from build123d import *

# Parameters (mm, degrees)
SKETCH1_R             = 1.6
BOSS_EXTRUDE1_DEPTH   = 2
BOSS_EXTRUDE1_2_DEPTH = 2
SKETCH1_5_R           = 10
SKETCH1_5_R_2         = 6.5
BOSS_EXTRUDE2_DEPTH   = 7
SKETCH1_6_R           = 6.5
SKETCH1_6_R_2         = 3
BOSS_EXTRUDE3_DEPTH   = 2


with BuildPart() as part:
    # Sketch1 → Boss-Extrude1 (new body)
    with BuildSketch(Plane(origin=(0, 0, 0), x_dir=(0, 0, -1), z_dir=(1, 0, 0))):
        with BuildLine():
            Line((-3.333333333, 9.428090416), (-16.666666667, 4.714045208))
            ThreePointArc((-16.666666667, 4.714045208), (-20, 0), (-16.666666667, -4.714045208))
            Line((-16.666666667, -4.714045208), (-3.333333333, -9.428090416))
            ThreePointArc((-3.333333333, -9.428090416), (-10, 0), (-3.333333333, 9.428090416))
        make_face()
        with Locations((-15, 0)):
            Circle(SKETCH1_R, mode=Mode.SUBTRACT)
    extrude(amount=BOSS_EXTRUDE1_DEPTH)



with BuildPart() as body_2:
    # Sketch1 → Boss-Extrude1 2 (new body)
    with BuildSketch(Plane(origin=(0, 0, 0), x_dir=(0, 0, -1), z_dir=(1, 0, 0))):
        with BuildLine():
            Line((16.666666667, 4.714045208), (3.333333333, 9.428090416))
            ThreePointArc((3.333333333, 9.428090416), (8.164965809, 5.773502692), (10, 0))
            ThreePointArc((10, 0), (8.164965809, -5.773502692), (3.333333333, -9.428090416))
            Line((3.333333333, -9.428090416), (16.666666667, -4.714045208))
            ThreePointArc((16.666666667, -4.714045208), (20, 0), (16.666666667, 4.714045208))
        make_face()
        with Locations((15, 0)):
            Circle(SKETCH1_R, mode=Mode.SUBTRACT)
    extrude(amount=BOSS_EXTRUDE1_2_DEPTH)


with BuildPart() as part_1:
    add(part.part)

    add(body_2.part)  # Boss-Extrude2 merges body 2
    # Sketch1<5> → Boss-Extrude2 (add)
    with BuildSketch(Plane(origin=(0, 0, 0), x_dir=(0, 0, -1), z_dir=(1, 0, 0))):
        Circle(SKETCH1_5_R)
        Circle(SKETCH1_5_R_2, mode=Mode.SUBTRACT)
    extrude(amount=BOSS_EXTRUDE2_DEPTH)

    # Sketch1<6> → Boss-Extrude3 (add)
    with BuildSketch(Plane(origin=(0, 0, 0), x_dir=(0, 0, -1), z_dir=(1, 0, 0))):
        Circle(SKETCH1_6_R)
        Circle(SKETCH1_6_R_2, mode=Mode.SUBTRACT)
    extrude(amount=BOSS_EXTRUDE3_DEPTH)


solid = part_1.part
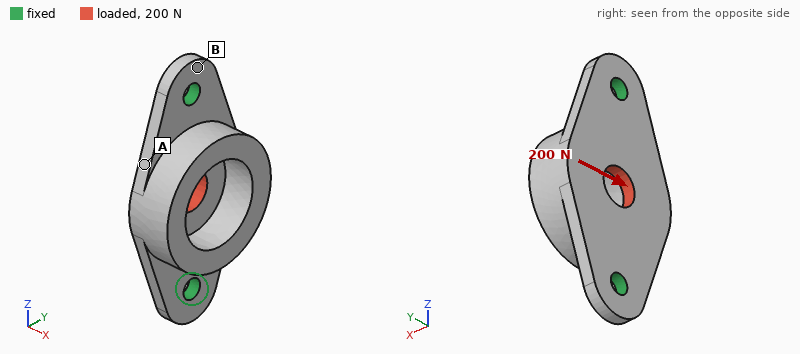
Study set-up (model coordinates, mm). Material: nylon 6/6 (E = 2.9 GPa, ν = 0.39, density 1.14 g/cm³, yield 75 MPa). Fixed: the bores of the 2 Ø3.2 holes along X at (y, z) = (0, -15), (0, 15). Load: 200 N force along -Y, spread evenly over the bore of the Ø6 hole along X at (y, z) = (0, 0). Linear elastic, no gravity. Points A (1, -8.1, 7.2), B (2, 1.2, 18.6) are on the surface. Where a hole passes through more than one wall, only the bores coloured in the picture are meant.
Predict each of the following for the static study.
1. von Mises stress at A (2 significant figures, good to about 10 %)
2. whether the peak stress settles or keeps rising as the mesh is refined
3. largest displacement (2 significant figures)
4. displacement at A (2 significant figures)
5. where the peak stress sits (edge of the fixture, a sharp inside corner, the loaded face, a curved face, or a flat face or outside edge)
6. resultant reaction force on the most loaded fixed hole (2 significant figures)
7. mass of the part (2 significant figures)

7.6 MPa
keeps rising
60 µm
40 µm
edge of the fixture
100 N
2.2 g
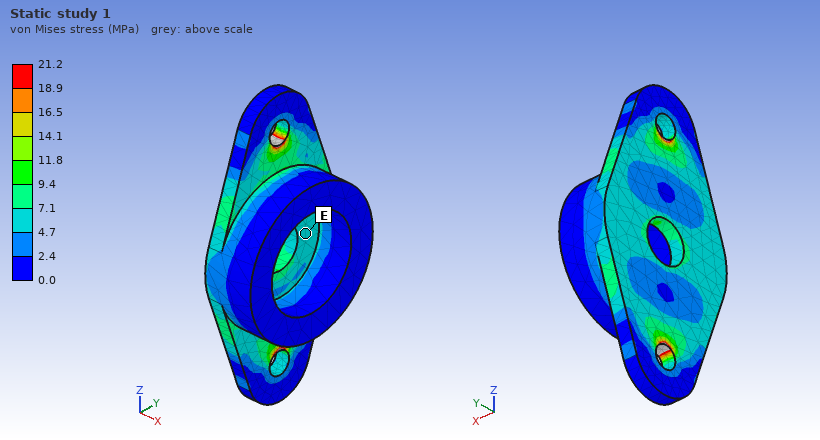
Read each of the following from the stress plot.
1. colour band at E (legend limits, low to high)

4.7 to 7.1 MPa
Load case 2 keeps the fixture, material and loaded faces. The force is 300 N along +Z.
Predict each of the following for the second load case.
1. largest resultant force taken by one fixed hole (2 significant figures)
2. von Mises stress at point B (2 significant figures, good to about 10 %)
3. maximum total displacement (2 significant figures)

150 N
2.9 MPa
35 µm
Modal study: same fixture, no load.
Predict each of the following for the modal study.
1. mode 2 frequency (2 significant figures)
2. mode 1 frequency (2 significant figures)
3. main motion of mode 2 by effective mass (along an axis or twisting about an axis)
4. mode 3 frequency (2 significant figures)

4100 Hz
2400 Hz
along X
9000 Hz
